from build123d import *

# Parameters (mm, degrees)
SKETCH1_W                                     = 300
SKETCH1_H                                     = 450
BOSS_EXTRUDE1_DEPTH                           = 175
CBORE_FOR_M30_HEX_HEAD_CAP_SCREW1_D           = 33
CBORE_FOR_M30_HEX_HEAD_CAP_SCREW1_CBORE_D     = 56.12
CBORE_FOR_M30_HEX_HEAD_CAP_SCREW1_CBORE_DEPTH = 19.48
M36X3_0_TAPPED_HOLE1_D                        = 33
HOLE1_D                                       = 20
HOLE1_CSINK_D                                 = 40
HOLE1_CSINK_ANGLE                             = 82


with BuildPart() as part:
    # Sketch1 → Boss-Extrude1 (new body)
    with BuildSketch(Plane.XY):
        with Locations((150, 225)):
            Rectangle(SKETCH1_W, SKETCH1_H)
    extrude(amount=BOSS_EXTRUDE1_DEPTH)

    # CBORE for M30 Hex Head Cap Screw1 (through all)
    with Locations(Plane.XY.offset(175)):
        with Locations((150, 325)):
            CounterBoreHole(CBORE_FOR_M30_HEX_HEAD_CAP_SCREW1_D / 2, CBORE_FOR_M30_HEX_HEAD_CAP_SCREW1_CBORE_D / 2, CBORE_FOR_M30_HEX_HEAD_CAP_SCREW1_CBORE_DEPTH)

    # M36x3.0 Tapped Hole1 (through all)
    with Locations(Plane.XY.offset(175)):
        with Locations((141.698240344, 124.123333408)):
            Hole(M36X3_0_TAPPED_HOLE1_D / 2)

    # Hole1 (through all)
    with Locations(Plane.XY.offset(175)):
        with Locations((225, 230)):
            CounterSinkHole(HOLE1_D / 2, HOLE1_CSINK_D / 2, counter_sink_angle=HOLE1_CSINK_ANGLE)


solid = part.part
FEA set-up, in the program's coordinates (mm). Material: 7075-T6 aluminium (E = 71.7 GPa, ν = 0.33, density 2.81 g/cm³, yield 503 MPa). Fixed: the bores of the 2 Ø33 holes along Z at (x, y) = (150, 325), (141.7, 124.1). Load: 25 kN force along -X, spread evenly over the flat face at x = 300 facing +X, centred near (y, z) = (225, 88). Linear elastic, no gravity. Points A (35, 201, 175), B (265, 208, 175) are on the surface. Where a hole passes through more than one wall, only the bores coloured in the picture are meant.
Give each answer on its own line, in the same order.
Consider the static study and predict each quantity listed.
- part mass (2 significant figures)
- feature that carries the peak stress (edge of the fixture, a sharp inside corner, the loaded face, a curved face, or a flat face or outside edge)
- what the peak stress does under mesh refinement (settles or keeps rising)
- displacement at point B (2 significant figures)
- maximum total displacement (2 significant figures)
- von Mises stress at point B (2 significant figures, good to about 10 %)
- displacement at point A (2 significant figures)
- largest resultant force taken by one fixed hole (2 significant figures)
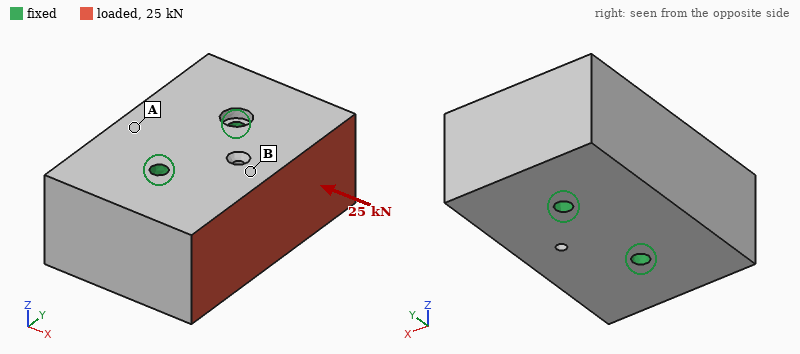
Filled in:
65 kg
edge of the fixture
keeps rising
0.82 µm
1.6 µm
0.35 MPa
0.27 µm
13 kN
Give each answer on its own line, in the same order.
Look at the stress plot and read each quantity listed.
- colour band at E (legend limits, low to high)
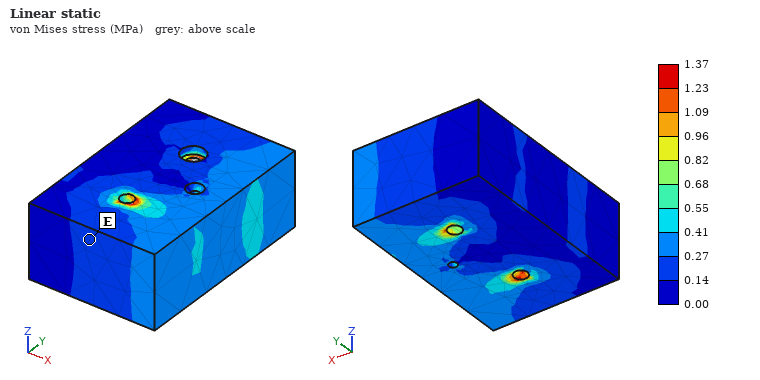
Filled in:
0.14 to 0.27 MPa
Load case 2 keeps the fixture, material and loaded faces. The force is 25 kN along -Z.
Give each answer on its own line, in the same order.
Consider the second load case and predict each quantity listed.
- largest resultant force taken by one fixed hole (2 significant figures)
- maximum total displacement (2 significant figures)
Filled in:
13 kN
8.2 µm
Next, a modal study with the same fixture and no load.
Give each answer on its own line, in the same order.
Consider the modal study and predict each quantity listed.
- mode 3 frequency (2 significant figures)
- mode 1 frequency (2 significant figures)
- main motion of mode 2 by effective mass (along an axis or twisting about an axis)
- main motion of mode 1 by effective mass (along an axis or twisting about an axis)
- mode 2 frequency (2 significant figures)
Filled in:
2800 Hz
2400 Hz
twisting about Z
twisting about Y
2500 Hz
